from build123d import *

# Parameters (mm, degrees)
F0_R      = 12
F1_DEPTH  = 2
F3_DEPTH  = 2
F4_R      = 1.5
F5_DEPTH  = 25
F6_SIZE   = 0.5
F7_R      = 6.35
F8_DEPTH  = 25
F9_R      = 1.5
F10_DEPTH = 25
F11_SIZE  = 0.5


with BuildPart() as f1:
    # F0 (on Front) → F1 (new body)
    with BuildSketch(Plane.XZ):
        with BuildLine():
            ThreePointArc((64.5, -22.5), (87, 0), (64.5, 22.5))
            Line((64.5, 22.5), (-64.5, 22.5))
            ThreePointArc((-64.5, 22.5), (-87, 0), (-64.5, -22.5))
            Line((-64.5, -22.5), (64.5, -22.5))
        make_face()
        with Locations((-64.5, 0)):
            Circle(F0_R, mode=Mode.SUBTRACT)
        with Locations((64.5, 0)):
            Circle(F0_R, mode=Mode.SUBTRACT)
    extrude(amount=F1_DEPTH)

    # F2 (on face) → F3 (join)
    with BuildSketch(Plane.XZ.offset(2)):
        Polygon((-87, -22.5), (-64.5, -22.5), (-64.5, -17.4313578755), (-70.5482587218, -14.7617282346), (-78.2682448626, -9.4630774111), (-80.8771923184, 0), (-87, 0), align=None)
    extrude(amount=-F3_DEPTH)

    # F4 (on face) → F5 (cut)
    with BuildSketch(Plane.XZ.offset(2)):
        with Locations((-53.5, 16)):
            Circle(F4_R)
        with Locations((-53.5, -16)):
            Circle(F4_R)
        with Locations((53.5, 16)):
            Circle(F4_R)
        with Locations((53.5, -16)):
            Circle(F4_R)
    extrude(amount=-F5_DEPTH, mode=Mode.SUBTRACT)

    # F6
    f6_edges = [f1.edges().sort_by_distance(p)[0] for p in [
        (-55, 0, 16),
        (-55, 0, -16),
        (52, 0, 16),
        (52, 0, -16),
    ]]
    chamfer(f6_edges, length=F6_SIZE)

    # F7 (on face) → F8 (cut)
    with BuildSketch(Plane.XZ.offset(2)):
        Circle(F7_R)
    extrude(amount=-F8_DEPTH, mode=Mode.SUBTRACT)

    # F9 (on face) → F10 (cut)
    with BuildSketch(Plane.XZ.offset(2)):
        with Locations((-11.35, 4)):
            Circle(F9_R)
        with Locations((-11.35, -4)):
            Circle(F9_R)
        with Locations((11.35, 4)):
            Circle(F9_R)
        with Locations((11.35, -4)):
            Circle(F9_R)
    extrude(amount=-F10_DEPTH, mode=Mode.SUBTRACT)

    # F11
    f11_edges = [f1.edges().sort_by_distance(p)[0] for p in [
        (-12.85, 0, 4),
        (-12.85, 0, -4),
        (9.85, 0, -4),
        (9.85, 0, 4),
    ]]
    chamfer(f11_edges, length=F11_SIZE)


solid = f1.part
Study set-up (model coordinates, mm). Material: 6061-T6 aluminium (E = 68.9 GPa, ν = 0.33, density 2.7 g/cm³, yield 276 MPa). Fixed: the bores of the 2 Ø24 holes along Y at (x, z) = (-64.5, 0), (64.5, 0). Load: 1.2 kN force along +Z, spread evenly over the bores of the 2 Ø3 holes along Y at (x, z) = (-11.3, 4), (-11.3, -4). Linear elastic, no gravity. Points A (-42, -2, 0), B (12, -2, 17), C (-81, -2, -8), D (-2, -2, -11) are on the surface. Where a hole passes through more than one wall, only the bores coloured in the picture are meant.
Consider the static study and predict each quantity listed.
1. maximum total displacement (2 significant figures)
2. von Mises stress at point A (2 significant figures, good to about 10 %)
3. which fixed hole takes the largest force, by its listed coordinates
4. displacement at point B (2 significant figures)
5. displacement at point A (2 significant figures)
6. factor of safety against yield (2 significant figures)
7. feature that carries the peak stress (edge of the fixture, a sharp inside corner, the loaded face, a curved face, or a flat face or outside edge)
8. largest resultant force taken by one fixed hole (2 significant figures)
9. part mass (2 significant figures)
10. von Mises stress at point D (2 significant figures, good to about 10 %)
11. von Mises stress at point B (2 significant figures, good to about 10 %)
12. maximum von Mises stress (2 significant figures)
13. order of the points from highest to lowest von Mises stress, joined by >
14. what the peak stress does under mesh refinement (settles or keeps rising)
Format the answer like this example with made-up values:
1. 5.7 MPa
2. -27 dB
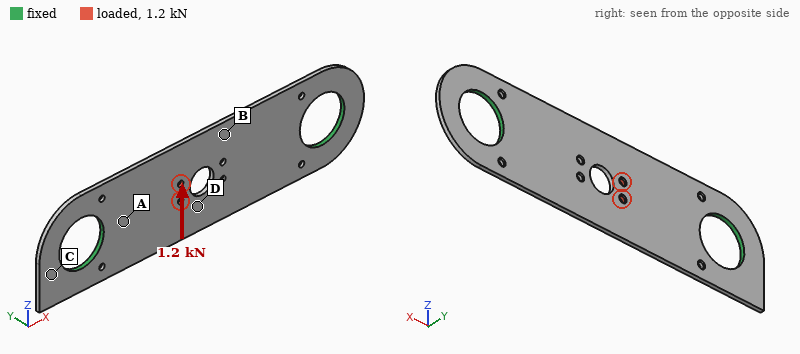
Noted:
1. 49 µm
2. 28 MPa
3. (-64.5, 0)
4. 31 µm
5. 9.3 µm
6. 3.5
7. the loaded face
8. 770 N
9. 35 g
10. 20 MPa
11. 11 MPa
12. 79 MPa
13. A > D > B > C
14. settles
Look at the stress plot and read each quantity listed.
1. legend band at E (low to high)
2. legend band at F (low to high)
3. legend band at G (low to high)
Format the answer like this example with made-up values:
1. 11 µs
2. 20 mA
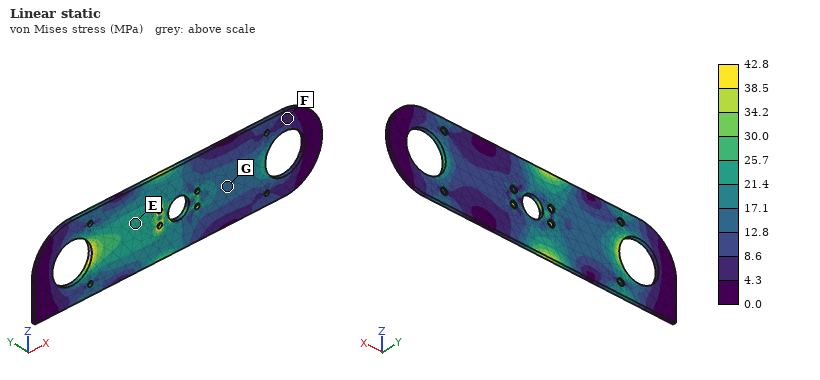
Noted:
1. 21.4 to 25.7 MPa
2. 4.3 to 8.6 MPa
3. 12.8 to 17.1 MPa
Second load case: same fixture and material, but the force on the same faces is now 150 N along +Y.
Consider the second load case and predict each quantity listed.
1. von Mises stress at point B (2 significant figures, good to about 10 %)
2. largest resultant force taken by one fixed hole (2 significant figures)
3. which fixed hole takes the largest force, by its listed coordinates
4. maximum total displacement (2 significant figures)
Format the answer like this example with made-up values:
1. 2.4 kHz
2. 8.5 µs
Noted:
1. 22 MPa
2. 98 N
3. (-64.5, 0)
4. 0.50 mm
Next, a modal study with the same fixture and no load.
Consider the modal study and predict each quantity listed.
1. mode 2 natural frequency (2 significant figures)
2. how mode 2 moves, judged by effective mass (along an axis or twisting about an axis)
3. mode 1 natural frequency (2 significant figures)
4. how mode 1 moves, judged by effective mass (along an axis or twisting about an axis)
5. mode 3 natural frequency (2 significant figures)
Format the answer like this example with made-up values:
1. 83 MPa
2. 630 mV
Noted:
1. 1400 Hz
2. twisting about X
3. 880 Hz
4. along Y
5. 2300 Hz
